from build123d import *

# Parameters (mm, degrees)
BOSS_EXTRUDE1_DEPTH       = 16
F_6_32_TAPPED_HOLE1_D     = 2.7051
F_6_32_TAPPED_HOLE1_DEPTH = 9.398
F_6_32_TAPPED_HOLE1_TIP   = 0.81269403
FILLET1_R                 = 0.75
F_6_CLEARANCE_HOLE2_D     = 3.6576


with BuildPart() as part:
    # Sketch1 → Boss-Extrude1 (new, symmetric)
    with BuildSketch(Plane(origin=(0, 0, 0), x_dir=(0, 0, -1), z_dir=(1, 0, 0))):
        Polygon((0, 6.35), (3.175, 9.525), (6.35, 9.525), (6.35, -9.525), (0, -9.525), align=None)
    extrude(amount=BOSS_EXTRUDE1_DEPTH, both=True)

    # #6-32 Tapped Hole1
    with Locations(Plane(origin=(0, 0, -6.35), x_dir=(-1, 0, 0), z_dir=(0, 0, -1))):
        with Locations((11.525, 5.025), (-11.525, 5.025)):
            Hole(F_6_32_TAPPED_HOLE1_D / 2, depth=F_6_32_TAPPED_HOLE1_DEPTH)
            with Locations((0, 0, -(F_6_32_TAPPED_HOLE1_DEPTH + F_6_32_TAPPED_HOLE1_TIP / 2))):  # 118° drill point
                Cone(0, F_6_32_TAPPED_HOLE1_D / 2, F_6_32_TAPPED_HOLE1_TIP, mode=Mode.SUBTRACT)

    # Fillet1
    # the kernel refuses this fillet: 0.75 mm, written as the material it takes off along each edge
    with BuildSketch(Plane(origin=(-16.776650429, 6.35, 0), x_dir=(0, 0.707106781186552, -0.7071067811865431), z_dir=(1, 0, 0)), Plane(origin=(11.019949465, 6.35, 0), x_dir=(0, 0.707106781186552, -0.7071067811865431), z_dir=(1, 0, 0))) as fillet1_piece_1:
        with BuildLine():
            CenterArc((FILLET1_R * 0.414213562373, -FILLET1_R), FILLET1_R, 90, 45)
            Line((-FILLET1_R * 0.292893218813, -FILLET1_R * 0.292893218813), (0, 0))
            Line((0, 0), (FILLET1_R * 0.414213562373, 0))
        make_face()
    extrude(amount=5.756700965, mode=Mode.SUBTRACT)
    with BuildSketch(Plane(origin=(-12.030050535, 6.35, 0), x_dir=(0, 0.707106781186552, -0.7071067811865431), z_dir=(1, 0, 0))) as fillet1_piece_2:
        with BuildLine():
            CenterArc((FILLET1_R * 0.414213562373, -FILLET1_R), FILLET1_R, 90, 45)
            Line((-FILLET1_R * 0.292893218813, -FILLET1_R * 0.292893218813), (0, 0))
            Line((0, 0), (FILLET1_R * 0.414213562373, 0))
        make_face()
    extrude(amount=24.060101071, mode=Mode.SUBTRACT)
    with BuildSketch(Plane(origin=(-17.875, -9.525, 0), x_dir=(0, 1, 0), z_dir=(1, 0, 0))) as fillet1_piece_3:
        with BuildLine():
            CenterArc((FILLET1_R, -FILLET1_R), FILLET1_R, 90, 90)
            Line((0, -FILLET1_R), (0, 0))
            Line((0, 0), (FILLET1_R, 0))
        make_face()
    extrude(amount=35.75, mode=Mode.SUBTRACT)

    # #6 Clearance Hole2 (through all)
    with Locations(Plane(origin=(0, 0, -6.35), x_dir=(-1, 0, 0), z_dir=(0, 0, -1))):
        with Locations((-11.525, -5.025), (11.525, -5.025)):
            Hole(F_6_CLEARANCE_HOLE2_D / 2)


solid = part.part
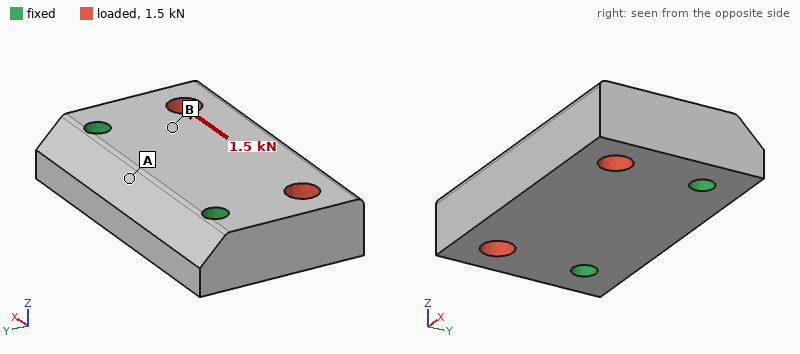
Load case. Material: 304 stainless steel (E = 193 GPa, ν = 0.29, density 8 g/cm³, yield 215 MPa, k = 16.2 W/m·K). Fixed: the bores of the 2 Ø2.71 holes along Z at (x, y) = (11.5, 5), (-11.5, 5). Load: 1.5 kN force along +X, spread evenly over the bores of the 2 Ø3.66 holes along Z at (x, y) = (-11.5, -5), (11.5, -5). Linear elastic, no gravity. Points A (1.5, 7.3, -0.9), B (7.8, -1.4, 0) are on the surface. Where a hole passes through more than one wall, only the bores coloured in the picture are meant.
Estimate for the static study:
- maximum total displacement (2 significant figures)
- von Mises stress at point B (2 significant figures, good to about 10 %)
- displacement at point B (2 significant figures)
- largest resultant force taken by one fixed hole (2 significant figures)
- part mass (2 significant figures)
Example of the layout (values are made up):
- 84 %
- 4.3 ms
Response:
- 2.2 µm
- 17 MPa
- 0.98 µm
- 950 N
- 28 g
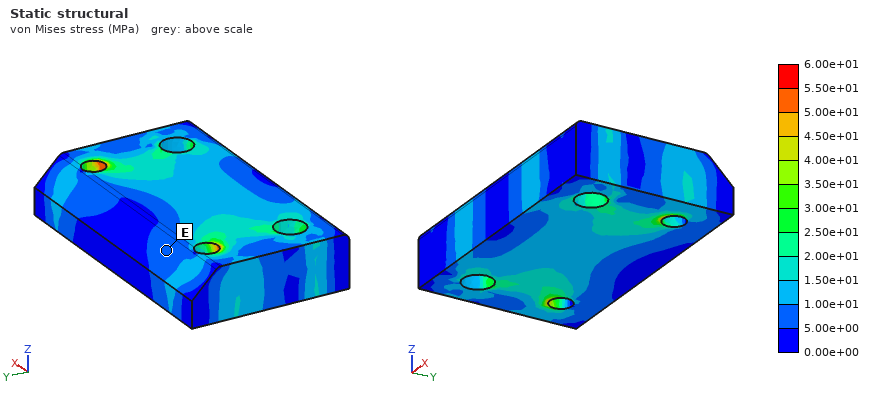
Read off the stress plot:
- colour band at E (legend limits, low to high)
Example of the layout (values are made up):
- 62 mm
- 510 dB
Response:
- 5.00e+00 to 1.00e+01 MPa
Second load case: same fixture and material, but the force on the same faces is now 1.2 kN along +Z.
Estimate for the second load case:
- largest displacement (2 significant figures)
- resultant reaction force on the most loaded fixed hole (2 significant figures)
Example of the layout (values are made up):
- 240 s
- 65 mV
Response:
- 9.9 µm
- 600 N
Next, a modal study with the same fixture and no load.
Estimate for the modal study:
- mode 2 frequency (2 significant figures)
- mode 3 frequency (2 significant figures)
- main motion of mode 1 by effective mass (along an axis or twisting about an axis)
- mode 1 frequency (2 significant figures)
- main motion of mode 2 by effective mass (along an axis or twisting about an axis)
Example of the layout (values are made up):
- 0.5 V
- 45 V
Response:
- 28 kHz
- 40 kHz
- along Z
- 17 kHz
- twisting about Y
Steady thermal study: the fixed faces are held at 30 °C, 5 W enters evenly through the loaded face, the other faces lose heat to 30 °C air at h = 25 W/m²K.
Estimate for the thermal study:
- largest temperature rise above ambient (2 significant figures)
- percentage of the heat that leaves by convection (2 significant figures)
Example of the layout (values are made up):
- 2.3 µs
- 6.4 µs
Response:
- 24 K
- 9.1 %
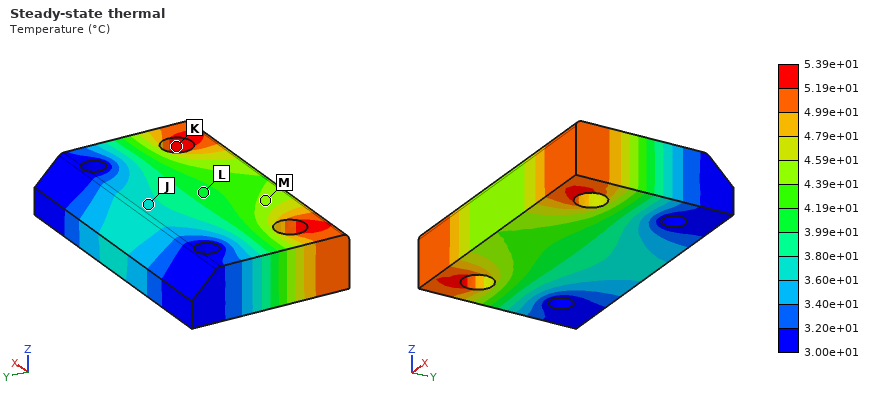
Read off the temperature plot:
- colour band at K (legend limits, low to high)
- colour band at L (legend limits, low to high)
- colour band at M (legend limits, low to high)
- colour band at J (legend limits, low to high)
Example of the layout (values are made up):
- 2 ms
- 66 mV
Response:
- 5.19e+01 to 5.39e+01 °C
- 3.99e+01 to 4.19e+01 °C
- 4.39e+01 to 4.59e+01 °C
- 3.60e+01 to 3.80e+01 °C
